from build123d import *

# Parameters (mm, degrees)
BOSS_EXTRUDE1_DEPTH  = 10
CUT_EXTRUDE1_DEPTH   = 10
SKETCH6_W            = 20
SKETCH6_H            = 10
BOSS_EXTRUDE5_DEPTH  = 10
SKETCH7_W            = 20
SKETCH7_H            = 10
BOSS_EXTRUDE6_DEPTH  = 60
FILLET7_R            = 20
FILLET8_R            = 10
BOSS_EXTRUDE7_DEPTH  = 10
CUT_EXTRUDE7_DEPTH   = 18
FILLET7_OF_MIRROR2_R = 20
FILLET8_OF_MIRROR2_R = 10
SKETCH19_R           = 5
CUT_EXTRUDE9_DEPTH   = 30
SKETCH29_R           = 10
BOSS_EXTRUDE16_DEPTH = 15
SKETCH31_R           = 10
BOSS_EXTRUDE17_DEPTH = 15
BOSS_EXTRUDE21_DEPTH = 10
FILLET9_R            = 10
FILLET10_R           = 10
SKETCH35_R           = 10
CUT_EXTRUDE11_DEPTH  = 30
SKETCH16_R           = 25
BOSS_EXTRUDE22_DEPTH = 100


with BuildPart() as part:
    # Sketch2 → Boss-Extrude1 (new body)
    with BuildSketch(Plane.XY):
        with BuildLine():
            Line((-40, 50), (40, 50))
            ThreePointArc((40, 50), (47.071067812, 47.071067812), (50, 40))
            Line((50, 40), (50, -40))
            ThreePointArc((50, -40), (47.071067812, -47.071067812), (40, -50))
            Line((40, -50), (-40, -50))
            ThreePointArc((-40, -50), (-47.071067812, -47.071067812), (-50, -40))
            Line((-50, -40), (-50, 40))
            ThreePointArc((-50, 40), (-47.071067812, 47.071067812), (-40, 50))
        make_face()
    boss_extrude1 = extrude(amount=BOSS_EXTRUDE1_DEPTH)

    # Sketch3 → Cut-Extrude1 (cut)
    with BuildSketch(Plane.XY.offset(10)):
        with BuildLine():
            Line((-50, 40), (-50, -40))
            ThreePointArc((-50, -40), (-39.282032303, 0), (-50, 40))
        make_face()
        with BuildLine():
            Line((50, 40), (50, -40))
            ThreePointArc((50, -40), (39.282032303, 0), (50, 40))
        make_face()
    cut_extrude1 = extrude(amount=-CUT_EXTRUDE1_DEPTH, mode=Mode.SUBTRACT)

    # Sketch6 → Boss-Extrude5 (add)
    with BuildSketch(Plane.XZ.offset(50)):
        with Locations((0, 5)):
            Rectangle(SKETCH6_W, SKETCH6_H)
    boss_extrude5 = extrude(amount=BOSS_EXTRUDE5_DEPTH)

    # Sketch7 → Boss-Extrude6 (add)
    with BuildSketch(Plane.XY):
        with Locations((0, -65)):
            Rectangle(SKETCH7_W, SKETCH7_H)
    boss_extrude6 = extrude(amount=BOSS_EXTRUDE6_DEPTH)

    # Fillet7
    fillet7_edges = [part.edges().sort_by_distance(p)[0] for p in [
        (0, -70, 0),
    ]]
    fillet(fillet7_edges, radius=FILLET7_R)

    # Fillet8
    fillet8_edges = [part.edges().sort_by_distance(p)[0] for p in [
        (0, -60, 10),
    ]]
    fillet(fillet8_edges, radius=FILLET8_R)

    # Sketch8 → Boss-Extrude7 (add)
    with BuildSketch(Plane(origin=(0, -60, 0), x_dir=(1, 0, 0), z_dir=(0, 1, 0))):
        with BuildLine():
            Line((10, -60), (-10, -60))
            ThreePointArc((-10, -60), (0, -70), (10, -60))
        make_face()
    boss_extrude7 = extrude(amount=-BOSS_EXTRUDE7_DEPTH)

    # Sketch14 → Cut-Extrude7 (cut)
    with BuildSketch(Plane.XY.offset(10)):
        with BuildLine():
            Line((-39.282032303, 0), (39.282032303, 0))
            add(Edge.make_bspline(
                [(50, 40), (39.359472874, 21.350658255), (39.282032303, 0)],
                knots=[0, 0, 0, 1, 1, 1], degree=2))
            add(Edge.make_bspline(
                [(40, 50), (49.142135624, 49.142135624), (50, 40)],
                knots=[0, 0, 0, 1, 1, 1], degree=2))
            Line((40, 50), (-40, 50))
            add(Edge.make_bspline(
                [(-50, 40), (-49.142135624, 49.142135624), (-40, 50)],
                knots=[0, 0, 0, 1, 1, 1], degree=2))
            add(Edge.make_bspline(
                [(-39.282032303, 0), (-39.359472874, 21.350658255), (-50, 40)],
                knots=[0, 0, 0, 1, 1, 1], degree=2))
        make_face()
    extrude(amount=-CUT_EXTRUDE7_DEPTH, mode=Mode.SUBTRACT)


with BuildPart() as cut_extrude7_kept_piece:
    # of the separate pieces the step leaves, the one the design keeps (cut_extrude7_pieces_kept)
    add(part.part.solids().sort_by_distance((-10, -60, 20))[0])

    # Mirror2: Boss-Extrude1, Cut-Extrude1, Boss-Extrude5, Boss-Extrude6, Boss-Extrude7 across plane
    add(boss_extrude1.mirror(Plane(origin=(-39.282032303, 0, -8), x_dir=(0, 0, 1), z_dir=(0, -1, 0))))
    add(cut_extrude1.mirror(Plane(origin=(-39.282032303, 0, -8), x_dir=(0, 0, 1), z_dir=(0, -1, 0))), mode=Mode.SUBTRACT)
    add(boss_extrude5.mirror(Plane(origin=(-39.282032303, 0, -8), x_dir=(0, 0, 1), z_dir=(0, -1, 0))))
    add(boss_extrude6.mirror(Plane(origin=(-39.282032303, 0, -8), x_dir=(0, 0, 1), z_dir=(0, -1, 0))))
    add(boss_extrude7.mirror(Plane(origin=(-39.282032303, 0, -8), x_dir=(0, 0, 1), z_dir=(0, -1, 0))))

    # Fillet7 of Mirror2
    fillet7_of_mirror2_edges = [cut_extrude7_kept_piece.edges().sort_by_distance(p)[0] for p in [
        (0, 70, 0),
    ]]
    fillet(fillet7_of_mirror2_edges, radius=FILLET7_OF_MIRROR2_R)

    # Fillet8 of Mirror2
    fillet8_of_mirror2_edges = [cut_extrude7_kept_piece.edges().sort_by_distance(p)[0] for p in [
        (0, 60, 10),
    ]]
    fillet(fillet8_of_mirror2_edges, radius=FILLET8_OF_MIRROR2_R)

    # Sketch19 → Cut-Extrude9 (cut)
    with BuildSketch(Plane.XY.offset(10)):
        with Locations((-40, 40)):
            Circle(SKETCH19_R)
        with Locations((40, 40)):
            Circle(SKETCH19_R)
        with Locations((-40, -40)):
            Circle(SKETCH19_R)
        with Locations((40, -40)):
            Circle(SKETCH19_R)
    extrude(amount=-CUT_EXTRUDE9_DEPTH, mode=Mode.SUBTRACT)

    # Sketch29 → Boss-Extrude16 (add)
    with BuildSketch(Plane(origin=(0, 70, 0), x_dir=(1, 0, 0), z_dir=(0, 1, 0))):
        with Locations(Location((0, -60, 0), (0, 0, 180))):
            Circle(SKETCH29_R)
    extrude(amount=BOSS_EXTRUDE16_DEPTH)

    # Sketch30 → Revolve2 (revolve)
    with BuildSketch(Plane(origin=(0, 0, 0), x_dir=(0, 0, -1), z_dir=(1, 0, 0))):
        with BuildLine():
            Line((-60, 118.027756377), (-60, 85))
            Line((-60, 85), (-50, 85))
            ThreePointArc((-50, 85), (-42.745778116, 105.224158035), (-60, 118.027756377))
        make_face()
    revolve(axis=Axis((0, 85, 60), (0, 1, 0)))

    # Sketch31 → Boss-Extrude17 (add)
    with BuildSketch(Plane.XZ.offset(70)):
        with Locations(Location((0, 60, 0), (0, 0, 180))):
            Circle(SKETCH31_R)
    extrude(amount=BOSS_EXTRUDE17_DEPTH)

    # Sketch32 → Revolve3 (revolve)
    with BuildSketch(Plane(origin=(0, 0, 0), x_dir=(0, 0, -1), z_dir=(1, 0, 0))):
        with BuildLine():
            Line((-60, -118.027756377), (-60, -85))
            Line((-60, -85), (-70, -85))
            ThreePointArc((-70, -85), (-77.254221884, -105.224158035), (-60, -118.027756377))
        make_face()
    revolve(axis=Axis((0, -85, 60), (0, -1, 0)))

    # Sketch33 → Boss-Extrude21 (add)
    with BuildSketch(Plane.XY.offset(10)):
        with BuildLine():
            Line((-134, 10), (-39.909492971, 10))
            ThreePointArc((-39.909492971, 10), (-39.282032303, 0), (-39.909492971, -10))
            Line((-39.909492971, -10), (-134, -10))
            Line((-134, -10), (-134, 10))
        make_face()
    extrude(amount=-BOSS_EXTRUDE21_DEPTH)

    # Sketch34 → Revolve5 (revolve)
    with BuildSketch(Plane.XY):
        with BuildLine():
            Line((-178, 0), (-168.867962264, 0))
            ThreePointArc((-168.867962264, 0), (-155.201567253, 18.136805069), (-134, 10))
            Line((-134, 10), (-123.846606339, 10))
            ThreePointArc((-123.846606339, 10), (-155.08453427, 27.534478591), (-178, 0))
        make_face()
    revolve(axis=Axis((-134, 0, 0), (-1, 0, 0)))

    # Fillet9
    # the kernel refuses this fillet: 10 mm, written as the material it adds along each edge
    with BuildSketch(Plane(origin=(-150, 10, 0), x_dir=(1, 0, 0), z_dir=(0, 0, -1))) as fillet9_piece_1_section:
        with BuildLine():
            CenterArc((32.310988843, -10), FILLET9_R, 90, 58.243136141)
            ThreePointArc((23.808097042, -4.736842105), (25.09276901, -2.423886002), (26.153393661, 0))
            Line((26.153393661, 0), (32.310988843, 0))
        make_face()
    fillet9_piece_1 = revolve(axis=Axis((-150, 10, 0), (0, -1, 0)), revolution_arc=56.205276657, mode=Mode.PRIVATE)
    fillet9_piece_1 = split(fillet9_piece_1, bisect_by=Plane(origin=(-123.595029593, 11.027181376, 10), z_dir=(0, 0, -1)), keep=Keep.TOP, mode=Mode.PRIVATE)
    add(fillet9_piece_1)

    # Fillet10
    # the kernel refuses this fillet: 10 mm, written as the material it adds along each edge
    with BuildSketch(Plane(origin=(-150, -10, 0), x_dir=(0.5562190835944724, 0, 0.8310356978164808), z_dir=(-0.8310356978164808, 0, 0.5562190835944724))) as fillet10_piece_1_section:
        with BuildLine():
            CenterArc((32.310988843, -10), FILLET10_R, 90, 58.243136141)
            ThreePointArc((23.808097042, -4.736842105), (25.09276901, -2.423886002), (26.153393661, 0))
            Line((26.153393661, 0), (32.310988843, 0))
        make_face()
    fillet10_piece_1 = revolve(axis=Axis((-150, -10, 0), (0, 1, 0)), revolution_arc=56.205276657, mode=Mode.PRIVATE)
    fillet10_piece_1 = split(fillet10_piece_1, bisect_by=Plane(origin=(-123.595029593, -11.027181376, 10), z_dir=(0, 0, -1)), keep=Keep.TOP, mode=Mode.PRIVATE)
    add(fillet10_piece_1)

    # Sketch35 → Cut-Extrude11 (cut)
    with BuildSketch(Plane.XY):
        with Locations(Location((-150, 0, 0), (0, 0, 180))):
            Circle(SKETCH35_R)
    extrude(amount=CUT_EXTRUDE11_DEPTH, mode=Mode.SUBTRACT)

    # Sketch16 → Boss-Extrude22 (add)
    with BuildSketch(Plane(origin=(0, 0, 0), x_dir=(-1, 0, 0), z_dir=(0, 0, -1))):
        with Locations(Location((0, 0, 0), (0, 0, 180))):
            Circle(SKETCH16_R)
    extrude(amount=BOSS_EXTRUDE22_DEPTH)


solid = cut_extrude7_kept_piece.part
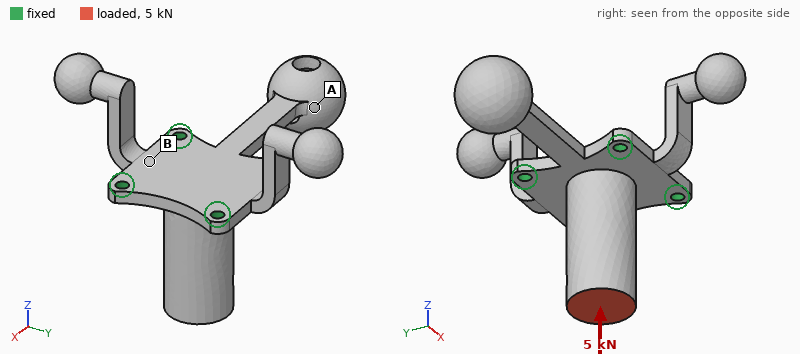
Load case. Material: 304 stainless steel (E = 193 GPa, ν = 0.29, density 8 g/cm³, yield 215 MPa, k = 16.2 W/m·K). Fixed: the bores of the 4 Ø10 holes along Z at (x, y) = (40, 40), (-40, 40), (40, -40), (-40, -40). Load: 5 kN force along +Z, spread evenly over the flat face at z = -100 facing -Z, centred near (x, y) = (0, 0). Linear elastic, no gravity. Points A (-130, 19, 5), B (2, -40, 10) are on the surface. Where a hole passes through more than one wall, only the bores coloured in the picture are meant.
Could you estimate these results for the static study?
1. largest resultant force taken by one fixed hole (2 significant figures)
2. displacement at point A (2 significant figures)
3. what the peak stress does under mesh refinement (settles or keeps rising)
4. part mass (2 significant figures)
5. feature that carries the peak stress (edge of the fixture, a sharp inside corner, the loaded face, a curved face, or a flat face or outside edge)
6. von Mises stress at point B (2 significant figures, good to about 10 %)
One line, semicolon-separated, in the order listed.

1.3 kN; 5.9 µm; keeps rising; 3.5 kg; edge of the fixture; 11 MPa
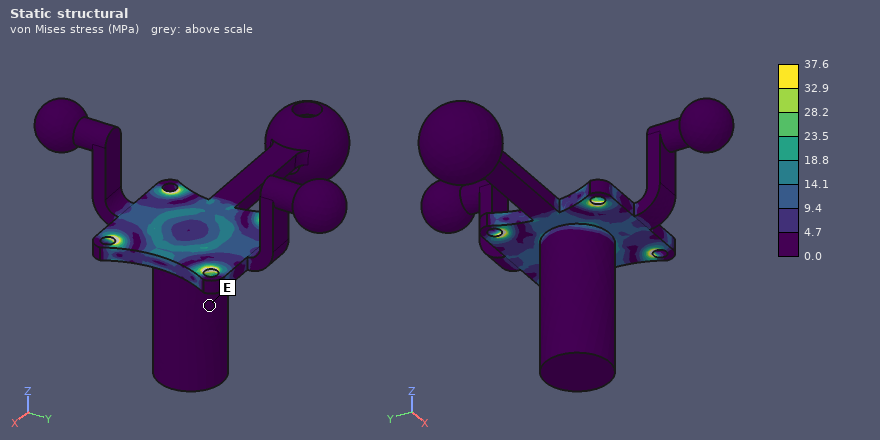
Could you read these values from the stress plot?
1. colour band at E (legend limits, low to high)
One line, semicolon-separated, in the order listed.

0.0 to 4.7 MPa
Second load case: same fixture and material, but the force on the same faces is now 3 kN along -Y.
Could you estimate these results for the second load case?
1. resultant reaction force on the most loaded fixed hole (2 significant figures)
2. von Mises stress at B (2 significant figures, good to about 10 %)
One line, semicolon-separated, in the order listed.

2.5 kN; 28 MPa
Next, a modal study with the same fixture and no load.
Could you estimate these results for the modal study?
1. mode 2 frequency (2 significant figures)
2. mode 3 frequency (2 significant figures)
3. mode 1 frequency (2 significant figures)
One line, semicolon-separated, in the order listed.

330 Hz; 370 Hz; 160 Hz
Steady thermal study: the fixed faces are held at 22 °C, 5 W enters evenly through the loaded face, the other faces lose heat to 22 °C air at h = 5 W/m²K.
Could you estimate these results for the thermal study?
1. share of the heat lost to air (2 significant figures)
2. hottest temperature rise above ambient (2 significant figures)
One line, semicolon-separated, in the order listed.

31 %; 20 K
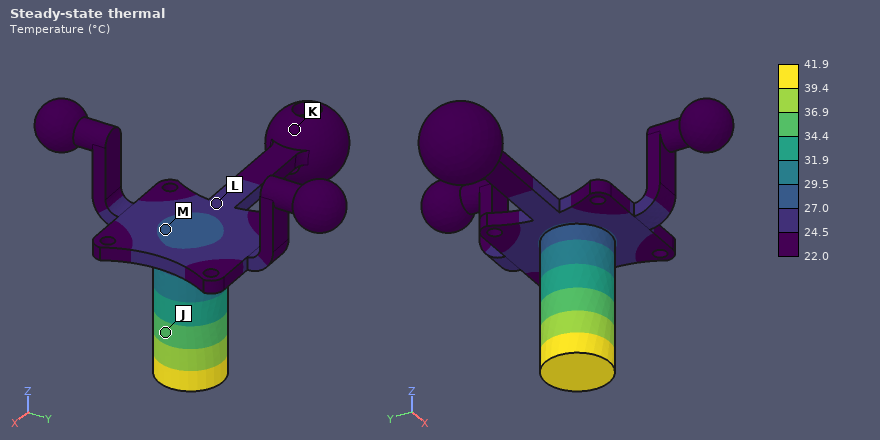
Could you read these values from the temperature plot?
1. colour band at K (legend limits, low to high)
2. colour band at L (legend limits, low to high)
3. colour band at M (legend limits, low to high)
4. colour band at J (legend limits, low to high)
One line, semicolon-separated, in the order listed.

22.0 to 24.5 °C; 24.5 to 27.0 °C; 27.0 to 29.5 °C; 34.4 to 36.9 °C
